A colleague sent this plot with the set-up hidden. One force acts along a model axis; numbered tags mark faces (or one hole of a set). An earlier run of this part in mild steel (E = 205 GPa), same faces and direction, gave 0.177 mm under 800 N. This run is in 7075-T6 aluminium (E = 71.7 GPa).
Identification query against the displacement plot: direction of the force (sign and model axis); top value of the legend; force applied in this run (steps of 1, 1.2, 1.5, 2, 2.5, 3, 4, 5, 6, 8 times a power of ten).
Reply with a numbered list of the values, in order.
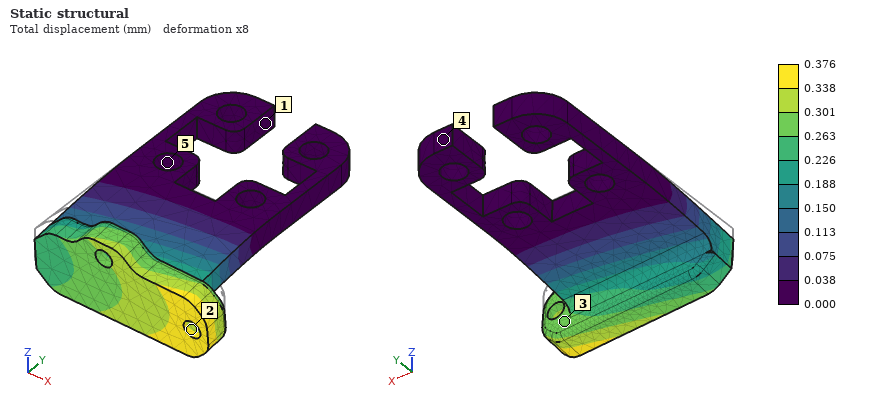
1. -Z
2. 0.376 mm
3. 600 N
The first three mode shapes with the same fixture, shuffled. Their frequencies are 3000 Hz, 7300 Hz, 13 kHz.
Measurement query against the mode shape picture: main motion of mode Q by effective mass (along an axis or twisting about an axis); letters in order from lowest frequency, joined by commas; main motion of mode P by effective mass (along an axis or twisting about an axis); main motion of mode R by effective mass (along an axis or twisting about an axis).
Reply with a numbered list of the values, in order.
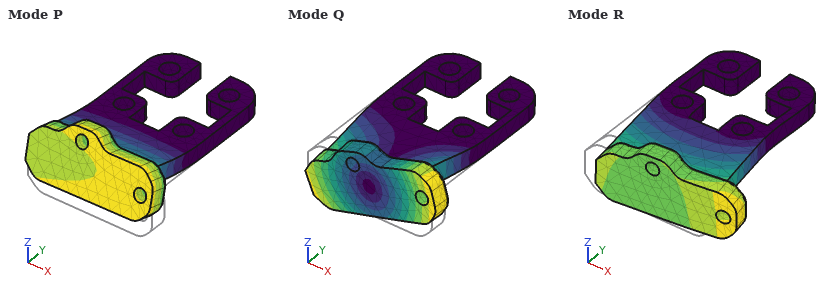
1. twisting about Y
2. P, Q, R
3. along Z
4. along X
